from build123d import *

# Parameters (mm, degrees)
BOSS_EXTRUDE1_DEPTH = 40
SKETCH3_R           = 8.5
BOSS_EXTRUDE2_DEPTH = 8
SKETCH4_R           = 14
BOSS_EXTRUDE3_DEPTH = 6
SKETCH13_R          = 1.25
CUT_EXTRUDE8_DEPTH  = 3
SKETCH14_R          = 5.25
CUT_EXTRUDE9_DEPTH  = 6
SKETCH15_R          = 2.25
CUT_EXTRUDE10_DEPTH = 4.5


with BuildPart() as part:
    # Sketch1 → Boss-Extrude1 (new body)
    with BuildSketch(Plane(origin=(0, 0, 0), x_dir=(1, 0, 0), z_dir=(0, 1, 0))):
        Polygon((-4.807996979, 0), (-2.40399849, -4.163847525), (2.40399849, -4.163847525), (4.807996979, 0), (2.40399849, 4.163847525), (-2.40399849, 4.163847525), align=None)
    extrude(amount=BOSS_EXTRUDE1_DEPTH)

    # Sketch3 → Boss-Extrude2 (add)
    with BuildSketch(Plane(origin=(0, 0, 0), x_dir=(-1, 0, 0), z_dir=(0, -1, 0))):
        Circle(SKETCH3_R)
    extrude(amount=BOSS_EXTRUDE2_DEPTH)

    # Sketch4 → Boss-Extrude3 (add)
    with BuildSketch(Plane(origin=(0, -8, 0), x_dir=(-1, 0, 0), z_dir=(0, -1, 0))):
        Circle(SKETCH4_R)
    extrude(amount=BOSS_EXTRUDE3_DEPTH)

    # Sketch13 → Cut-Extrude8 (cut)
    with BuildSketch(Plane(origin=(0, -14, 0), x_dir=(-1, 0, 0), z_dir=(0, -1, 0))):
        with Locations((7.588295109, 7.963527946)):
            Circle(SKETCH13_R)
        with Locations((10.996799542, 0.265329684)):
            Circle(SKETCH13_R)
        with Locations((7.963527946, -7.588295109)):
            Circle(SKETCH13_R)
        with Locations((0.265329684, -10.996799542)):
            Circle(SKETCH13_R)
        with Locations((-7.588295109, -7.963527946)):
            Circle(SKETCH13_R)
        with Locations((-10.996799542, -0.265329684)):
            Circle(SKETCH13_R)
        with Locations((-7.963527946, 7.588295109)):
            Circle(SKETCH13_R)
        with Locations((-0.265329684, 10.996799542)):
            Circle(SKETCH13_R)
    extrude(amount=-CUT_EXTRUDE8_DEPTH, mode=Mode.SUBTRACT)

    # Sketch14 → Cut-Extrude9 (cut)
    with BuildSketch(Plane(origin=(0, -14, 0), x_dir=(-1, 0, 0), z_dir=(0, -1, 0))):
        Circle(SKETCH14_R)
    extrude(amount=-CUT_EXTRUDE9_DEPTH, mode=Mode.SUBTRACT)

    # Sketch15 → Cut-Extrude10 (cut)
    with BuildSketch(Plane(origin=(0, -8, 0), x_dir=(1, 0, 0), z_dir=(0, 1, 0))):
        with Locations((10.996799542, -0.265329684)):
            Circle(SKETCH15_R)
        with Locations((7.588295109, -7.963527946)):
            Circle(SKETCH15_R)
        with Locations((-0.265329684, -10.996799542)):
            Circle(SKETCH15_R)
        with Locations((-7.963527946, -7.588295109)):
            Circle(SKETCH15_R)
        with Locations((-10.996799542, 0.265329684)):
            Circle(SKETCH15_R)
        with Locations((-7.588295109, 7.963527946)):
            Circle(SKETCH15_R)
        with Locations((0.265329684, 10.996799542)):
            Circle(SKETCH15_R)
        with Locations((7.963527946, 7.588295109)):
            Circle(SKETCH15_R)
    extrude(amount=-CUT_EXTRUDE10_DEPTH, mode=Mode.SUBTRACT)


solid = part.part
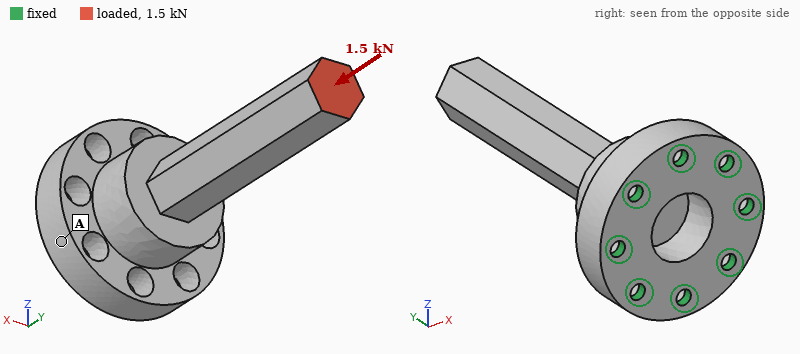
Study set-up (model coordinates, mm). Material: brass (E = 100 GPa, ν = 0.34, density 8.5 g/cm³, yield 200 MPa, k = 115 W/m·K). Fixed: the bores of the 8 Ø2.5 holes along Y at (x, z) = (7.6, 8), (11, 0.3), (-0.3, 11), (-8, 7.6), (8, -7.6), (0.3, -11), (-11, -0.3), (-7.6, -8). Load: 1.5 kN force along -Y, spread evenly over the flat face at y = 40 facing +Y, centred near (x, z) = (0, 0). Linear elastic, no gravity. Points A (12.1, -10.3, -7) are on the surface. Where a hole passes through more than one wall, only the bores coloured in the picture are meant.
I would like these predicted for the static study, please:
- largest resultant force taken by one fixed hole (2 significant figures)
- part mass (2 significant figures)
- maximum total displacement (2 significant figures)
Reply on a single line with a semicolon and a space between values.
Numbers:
220 N; 57 g; 13 µm
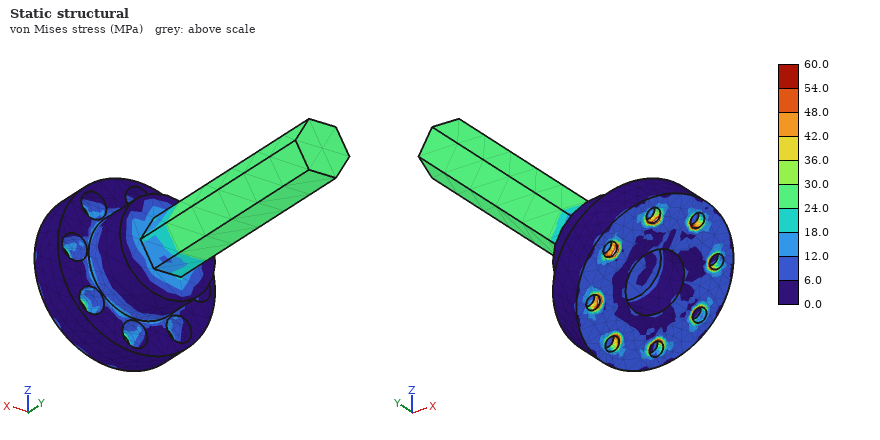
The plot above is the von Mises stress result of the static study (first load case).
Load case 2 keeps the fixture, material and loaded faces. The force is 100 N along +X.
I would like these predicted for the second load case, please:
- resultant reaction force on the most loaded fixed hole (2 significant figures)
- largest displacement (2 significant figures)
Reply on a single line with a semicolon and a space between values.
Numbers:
130 N; 94 µm
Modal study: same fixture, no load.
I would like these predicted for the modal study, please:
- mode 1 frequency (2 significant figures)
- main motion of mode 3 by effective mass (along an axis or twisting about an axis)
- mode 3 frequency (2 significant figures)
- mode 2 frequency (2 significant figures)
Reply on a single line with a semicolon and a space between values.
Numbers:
2200 Hz; along Z; 11 kHz; 2200 Hz
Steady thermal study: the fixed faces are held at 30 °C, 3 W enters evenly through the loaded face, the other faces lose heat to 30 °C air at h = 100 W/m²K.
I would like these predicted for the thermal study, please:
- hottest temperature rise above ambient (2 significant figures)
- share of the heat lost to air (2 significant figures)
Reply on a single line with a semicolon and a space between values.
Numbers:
16 K; 36 %
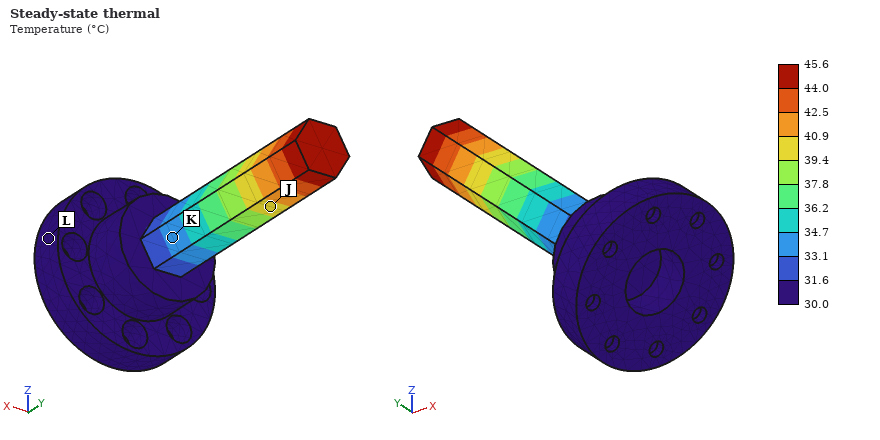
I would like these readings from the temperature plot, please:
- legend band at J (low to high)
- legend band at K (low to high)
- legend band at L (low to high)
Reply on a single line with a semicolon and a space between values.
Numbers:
39.4 to 40.9 °C; 33.1 to 34.7 °C; 30.0 to 31.6 °C
